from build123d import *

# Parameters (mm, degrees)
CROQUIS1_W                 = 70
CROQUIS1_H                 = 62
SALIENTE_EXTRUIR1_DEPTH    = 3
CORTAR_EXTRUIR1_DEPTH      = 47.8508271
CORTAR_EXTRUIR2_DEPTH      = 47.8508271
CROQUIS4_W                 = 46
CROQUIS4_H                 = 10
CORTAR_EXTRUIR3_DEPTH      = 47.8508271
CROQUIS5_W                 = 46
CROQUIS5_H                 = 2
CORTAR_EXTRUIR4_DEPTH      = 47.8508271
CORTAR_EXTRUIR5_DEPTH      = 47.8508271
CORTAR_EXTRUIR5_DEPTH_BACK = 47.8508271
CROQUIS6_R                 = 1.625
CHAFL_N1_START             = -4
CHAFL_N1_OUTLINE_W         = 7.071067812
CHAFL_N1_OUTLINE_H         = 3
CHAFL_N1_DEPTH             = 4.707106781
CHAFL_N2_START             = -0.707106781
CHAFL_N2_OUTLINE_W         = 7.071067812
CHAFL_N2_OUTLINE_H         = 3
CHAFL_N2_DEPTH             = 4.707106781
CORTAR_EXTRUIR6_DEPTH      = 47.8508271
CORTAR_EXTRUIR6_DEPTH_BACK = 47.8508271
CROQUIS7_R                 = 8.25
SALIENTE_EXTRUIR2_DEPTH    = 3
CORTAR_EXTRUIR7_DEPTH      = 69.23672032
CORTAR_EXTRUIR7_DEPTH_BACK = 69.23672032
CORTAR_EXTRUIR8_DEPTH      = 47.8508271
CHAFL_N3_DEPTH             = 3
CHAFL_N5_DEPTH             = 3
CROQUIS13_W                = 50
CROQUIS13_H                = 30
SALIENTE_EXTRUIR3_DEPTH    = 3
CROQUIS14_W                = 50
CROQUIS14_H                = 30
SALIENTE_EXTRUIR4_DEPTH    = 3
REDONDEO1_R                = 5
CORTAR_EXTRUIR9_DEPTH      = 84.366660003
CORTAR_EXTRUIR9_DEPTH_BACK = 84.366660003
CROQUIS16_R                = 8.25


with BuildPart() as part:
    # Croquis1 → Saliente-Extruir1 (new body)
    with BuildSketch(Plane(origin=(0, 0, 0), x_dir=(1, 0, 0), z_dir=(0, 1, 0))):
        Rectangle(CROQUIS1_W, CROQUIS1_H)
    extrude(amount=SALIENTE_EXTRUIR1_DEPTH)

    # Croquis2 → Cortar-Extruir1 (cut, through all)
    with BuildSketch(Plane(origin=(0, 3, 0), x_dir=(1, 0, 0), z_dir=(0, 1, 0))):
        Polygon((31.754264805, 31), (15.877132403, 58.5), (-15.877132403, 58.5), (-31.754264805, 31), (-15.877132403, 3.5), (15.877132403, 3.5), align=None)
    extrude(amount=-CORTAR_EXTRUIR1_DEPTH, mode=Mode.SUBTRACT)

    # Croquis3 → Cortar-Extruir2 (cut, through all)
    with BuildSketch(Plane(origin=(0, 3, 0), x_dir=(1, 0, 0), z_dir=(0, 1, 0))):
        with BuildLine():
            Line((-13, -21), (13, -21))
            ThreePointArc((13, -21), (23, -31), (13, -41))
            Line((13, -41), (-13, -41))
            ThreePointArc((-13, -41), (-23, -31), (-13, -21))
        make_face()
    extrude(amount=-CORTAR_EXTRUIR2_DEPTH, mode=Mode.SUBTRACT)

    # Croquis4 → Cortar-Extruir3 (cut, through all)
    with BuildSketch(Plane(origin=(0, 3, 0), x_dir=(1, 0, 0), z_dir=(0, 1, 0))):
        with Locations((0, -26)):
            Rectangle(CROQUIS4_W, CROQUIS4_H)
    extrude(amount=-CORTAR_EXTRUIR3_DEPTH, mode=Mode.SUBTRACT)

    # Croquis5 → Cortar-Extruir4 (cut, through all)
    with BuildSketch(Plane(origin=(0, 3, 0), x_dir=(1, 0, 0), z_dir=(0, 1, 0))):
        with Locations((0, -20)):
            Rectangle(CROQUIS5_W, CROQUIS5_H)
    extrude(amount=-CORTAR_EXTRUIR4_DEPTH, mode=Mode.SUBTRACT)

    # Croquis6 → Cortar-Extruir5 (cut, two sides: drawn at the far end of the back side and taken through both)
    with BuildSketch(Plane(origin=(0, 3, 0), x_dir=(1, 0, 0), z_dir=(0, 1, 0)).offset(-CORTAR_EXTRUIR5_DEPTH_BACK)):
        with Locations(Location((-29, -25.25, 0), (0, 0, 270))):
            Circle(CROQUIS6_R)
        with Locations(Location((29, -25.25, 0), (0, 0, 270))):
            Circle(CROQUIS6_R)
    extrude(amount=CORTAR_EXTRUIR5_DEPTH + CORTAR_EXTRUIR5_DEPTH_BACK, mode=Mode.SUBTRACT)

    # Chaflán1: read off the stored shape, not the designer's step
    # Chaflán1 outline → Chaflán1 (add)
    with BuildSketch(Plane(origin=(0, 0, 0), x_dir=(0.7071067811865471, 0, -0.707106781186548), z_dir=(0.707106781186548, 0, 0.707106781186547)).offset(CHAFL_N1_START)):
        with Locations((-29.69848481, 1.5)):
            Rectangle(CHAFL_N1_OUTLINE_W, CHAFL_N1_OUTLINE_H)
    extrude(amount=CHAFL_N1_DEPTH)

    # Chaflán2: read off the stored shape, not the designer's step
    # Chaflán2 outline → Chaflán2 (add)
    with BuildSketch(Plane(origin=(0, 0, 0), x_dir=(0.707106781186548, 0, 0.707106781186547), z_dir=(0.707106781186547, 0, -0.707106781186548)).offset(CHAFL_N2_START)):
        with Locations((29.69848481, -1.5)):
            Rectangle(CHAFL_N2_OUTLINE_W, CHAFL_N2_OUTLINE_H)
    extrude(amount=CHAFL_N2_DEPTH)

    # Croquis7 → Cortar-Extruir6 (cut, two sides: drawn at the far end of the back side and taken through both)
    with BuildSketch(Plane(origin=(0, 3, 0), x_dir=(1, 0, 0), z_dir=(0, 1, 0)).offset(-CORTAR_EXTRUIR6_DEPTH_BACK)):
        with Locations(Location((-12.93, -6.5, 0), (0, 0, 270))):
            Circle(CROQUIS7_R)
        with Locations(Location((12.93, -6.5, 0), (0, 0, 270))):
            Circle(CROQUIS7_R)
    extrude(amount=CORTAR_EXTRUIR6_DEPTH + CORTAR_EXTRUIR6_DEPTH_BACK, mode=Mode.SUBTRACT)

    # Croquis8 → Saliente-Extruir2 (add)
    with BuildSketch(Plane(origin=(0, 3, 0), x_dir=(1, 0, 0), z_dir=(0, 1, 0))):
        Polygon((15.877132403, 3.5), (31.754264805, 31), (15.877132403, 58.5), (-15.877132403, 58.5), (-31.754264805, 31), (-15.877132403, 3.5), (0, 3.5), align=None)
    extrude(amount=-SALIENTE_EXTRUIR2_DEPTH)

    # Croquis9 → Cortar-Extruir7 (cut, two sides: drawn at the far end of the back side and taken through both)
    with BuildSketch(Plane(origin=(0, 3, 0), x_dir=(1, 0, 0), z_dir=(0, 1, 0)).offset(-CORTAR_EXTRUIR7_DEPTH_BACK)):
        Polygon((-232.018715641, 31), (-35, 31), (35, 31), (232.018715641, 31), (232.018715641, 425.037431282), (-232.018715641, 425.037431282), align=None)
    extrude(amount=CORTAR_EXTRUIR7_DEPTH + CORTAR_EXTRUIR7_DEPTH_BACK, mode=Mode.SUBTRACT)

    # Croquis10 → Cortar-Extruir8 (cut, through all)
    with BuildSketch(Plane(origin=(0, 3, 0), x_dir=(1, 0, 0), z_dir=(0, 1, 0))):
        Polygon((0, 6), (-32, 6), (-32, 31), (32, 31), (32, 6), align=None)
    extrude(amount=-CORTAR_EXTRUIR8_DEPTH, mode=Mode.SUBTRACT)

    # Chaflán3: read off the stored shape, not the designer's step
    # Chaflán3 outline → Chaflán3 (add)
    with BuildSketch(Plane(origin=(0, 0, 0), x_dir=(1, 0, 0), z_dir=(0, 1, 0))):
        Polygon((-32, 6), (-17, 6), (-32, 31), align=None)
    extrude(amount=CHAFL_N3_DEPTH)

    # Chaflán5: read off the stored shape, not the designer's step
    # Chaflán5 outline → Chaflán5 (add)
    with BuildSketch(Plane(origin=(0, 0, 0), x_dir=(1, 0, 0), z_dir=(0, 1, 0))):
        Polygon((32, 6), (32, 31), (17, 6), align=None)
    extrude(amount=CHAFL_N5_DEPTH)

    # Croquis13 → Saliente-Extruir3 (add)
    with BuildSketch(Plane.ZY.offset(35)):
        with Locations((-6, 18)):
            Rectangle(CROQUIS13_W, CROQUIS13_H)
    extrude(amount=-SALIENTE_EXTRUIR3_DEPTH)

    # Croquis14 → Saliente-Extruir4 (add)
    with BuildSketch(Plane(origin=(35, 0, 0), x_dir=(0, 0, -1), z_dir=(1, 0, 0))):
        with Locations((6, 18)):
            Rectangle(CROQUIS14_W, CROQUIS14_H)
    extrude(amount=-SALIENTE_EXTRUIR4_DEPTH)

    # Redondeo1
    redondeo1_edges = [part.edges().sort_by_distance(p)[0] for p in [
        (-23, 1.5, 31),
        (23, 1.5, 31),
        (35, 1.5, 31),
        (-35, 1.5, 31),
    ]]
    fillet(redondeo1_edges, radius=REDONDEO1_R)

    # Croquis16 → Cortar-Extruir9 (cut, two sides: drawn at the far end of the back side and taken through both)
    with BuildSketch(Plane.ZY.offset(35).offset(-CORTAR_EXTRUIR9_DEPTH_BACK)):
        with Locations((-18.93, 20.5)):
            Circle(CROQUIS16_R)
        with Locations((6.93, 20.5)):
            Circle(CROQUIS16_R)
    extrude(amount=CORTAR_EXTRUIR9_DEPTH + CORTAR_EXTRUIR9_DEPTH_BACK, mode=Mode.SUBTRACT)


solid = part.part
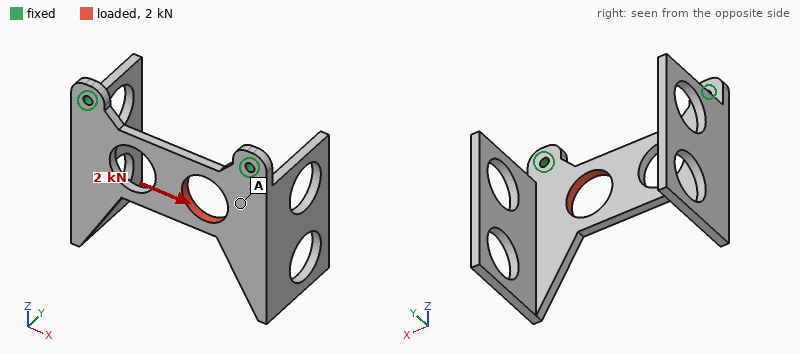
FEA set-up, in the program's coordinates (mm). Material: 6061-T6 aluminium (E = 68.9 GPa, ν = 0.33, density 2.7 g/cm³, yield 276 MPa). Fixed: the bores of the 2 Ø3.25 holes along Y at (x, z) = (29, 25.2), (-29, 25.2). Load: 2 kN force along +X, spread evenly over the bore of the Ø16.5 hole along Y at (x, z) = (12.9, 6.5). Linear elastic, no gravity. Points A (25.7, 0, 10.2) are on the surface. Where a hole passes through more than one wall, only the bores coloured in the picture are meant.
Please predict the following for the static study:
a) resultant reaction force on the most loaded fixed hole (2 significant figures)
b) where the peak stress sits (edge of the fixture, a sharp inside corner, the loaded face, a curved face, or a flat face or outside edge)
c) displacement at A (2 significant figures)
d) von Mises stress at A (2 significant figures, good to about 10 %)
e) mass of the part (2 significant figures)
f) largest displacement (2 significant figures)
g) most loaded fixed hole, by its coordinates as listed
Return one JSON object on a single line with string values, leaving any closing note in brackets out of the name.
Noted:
{"resultant reaction force on the most loaded fixed hole": "1.2 kN", "where the peak stress sits": "edge of the fixture", "displacement at A": "37 µm", "von Mises stress at A": "20 MPa", "mass of the part": "35 g", "largest displacement": "99 µm", "most loaded fixed hole, by its coordinates as listed": "(29, 25.2)"}
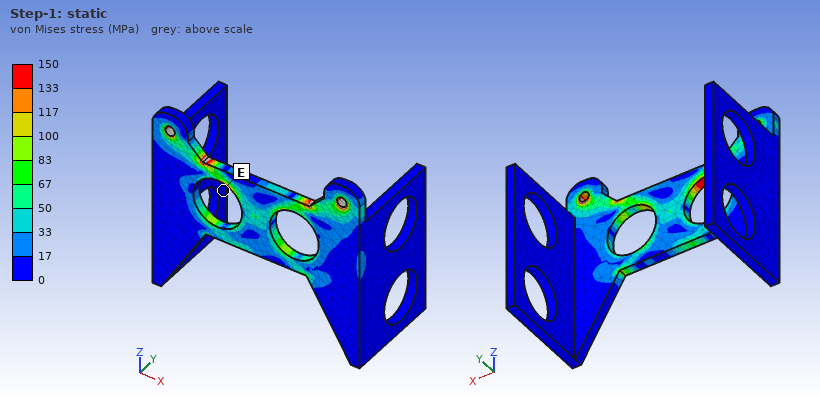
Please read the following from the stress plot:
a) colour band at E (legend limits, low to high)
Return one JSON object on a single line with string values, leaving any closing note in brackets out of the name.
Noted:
{"colour band at E": "0 to 17 MPa"}
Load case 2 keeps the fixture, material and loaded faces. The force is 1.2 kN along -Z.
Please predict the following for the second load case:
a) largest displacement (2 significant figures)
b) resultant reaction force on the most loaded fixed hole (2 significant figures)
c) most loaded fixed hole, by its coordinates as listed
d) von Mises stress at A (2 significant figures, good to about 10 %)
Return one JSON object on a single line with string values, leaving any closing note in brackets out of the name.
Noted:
{"largest displacement": "33 µm", "resultant reaction force on the most loaded fixed hole": "940 N", "most loaded fixed hole, by its coordinates as listed": "(29, 25.2)", "von Mises stress at A": "28 MPa"}
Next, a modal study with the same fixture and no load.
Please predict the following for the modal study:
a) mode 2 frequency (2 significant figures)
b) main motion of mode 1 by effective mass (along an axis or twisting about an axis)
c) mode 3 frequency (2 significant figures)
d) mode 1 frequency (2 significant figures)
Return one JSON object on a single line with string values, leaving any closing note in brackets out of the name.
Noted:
{"mode 2 frequency": "720 Hz", "main motion of mode 1 by effective mass": "along Y", "mode 3 frequency": "1200 Hz", "mode 1 frequency": "610 Hz"}
